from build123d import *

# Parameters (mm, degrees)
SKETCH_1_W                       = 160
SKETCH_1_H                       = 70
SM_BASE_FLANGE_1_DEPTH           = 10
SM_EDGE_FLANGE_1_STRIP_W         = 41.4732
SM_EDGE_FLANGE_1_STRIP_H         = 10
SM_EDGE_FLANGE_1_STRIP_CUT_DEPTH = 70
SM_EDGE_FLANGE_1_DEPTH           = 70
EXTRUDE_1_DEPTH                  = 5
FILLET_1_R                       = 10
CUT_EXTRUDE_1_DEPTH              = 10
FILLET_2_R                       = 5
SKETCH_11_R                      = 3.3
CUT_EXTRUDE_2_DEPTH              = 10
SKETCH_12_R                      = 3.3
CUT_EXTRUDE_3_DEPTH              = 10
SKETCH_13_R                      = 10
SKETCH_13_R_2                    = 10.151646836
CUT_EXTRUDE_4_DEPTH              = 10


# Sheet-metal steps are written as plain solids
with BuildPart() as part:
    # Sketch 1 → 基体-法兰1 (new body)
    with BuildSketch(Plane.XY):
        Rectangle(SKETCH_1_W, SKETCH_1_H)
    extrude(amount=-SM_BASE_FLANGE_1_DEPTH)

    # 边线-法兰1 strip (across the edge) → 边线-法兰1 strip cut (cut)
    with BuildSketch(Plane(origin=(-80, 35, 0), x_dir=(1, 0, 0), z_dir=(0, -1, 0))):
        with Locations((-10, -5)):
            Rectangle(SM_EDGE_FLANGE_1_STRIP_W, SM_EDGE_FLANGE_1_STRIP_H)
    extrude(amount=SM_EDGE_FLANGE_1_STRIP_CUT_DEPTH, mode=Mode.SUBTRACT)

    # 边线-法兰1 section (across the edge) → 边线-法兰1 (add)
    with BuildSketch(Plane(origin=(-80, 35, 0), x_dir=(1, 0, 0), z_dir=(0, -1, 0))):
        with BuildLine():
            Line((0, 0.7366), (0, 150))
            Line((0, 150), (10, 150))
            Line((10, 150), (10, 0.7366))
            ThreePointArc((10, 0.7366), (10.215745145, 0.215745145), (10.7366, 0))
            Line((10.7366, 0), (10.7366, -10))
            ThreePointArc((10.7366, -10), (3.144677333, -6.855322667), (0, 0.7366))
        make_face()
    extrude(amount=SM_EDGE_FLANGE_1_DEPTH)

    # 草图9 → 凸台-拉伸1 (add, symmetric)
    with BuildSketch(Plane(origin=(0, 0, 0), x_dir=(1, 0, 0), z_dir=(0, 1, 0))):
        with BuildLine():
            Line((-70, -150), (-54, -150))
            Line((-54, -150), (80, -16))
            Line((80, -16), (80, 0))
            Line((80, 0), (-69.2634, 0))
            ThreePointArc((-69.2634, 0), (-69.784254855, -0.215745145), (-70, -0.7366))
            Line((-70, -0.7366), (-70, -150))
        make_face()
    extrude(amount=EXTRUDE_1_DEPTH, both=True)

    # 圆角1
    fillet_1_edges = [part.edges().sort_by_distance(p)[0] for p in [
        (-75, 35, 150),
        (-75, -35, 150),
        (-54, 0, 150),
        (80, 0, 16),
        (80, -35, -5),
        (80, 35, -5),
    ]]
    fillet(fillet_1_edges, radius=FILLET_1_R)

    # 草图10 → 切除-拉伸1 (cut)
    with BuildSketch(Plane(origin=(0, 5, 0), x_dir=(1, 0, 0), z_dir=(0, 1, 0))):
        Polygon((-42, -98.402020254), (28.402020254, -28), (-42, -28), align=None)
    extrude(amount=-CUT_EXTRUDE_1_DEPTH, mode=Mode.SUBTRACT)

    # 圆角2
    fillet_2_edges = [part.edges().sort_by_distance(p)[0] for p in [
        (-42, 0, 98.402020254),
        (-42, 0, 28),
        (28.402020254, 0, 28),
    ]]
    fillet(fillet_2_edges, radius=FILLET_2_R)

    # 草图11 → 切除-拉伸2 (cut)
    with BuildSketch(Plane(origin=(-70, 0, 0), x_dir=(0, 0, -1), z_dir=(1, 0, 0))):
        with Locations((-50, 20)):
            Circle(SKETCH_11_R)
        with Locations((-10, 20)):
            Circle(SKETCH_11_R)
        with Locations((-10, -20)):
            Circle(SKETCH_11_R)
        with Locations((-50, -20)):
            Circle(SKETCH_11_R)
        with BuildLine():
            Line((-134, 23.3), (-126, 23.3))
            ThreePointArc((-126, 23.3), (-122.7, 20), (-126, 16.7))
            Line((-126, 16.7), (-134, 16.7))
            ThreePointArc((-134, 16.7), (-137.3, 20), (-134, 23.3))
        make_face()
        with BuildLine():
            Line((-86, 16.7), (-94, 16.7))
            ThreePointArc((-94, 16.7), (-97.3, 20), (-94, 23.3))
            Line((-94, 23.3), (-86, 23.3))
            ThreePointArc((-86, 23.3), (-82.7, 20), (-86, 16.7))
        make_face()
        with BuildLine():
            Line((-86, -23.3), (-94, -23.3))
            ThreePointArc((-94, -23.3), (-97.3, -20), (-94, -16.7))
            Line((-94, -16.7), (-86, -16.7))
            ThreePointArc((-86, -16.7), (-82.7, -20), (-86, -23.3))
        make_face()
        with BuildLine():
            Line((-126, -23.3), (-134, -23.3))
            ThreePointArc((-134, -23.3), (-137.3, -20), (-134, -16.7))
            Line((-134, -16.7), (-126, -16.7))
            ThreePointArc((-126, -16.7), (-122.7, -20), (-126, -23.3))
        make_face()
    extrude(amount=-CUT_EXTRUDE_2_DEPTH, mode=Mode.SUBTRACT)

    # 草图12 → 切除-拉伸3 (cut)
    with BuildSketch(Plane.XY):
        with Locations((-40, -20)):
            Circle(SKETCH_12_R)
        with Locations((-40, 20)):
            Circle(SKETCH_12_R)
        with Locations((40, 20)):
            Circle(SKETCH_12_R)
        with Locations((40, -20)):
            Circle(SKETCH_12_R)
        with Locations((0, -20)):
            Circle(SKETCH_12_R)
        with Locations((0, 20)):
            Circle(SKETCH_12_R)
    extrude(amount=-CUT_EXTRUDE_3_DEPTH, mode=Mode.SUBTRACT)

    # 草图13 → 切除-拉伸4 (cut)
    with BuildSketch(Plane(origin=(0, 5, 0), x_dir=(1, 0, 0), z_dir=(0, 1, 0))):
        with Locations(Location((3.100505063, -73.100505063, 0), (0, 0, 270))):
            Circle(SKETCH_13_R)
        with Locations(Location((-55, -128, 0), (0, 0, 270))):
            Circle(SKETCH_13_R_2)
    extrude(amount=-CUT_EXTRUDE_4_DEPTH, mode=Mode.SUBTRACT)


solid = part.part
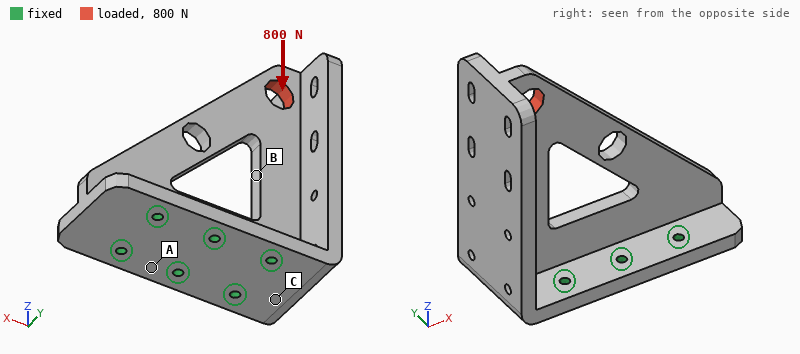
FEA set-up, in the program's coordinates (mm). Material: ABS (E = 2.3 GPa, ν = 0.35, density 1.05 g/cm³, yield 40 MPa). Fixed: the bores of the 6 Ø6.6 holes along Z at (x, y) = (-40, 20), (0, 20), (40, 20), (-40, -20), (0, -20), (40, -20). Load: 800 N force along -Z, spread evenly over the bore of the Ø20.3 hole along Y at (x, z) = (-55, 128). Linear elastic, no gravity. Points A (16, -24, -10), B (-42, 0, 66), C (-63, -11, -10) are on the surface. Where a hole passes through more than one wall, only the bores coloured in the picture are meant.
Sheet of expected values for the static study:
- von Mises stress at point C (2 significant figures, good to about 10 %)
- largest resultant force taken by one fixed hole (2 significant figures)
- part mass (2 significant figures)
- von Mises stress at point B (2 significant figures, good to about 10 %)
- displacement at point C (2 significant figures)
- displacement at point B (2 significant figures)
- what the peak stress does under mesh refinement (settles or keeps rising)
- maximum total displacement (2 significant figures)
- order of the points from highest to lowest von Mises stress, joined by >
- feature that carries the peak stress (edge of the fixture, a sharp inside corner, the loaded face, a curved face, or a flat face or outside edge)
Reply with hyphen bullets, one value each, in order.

- 1.1 MPa
- 440 N
- 330 g
- 2.8 MPa
- 0.12 mm
- 0.20 mm
- keeps rising
- 0.31 mm
- B > C > A
- edge of the fixture
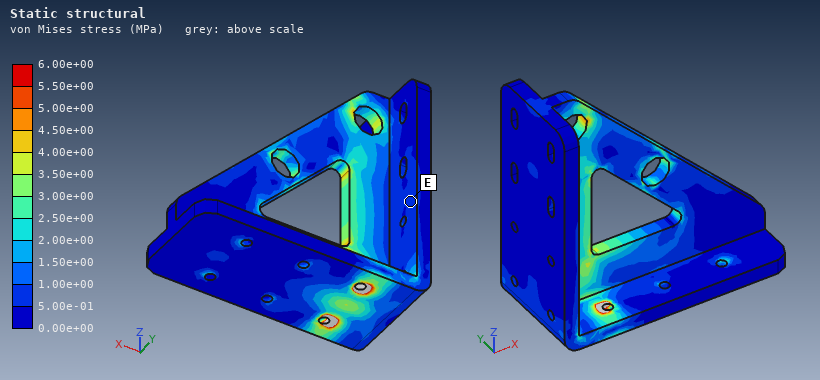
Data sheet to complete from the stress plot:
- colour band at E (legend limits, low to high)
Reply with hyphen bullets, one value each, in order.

- 5.00e-01 to 1.00e+00 MPa
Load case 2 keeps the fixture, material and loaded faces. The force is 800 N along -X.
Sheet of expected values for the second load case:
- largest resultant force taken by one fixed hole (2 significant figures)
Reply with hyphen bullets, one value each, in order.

- 610 N
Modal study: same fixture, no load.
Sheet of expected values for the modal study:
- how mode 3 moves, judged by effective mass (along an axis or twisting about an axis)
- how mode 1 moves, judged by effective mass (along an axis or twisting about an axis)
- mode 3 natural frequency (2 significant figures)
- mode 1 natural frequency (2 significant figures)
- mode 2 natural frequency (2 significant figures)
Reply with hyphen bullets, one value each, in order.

- along X
- along Y
- 470 Hz
- 190 Hz
- 430 Hz
